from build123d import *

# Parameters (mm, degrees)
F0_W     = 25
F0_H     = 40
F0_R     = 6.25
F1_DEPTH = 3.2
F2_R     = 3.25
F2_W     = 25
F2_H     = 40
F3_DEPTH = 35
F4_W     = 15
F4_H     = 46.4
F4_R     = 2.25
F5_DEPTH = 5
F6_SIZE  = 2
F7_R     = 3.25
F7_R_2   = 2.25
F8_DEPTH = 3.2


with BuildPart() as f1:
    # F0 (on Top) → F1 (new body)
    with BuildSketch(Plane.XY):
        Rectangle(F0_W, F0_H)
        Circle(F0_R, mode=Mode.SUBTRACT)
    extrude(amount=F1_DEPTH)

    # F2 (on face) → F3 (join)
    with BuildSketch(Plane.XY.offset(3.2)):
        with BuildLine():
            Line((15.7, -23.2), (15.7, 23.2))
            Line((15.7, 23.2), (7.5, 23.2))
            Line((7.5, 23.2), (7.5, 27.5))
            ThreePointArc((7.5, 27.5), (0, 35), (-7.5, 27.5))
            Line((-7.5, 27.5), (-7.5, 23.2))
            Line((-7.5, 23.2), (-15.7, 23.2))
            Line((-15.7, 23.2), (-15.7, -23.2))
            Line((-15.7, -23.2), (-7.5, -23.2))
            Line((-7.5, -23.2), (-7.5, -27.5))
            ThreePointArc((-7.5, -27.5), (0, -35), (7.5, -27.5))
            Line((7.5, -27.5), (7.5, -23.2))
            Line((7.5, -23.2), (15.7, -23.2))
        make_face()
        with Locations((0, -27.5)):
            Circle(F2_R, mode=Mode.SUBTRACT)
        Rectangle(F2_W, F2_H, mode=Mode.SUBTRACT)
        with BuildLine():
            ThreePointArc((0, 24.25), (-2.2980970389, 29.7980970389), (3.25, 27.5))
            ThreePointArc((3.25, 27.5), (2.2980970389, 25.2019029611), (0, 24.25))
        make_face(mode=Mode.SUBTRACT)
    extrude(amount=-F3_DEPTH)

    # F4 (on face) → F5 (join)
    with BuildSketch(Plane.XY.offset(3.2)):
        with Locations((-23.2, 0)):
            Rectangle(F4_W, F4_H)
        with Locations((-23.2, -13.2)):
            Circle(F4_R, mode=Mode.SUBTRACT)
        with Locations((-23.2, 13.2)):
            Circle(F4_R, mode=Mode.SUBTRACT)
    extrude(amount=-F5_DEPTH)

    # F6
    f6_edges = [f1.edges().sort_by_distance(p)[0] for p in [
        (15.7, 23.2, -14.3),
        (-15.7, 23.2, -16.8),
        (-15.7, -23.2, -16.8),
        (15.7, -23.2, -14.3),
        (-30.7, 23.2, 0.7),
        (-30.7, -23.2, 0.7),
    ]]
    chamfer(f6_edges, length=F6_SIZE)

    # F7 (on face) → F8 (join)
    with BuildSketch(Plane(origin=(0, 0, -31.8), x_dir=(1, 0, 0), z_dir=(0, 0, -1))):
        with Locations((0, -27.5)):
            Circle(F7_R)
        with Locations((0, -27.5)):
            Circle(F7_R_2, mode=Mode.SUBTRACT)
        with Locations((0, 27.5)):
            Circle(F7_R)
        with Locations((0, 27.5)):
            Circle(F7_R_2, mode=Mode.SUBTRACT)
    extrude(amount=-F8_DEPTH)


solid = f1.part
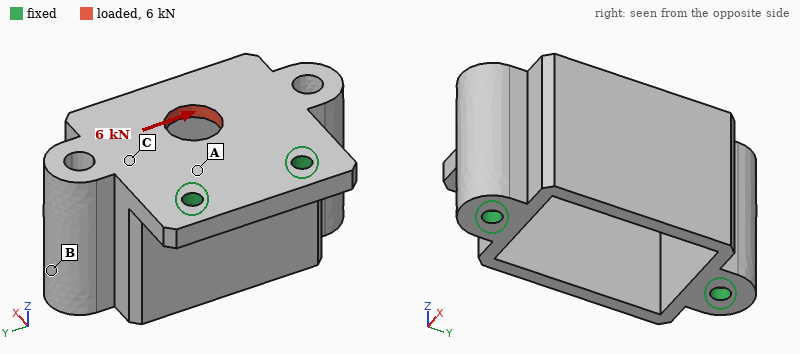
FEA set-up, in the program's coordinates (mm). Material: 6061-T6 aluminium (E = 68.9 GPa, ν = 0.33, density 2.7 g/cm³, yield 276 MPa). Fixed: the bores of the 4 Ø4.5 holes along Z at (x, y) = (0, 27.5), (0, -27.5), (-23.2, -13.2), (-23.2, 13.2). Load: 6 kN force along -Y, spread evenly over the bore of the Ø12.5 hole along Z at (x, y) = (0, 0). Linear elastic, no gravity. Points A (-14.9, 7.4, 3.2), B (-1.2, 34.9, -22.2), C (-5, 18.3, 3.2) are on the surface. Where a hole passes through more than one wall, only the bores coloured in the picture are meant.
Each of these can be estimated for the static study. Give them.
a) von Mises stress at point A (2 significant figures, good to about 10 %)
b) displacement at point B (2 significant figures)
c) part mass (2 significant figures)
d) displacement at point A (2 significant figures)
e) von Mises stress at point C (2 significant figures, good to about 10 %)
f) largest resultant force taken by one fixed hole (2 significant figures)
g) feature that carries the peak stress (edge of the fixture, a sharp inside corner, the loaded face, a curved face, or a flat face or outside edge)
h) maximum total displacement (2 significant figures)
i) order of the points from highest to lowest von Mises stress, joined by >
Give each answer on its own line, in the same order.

48 MPa
16 µm
82 g
9.0 µm
26 MPa
2.8 kN
edge of the fixture
44 µm
A > C > B
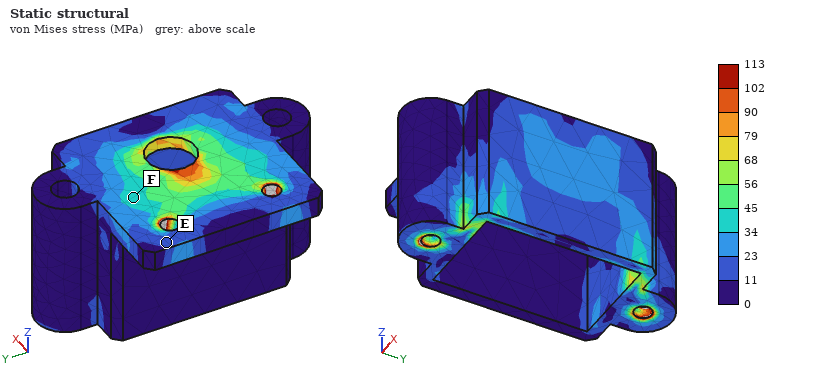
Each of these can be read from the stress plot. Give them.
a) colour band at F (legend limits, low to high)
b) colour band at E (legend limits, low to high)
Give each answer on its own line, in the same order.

34 to 45 MPa
11 to 23 MPa
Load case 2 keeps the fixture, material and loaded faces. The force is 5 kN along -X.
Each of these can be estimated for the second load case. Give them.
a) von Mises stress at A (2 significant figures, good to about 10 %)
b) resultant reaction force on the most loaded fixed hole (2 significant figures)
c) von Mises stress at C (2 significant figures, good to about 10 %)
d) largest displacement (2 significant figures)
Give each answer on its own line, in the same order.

43 MPa
2.5 kN
15 MPa
25 µm
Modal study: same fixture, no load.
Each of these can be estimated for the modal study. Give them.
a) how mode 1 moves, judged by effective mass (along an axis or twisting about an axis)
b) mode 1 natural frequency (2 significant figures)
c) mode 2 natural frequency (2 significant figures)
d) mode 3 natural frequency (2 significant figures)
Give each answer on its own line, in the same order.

along Y
8200 Hz
8700 Hz
9100 Hz
